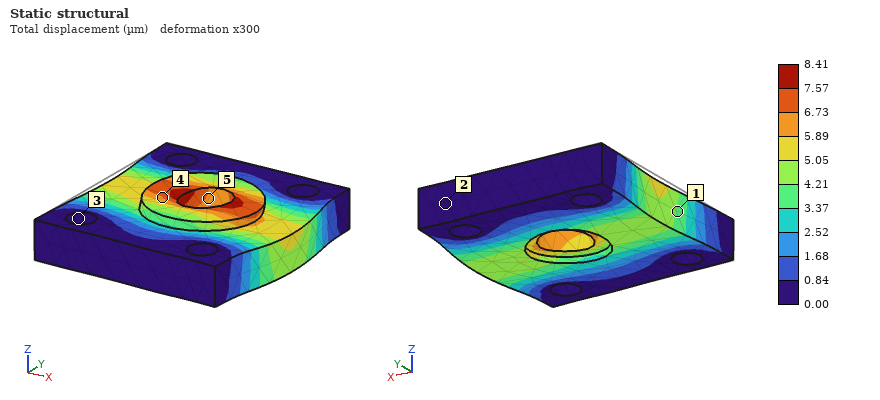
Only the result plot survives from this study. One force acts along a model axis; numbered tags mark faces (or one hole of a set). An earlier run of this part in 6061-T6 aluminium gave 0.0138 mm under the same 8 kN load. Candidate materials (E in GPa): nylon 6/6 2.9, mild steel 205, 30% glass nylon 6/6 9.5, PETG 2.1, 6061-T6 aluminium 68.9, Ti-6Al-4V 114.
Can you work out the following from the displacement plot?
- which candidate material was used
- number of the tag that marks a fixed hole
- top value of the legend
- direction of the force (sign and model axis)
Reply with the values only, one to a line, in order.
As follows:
Ti-6Al-4V
3
8.41 µm
+X
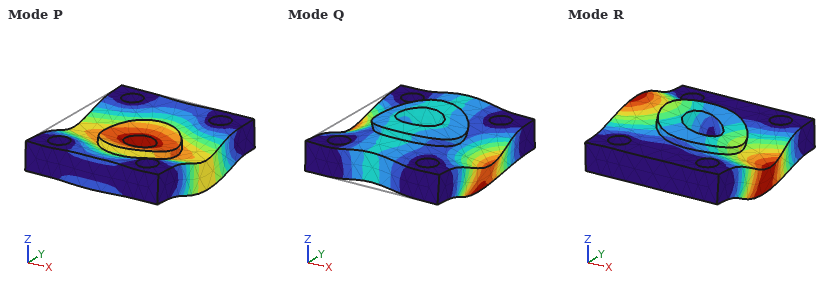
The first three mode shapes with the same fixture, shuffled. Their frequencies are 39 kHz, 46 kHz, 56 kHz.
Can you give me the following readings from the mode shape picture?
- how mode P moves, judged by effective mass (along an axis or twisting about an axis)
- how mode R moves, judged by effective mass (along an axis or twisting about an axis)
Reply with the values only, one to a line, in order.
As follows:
along Z
twisting about Y
